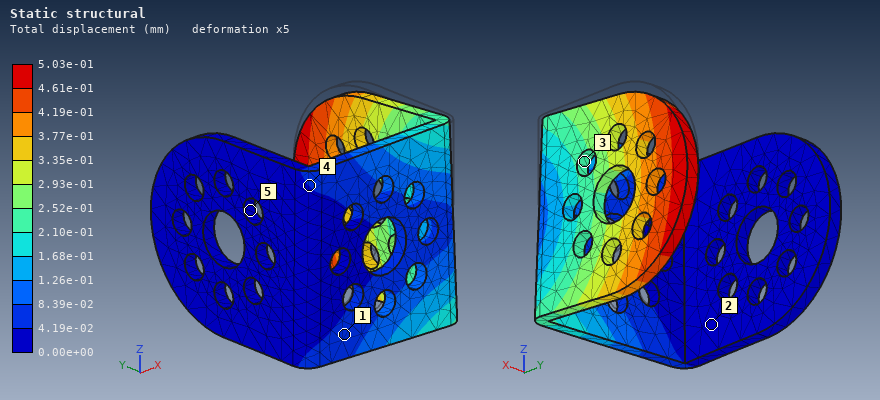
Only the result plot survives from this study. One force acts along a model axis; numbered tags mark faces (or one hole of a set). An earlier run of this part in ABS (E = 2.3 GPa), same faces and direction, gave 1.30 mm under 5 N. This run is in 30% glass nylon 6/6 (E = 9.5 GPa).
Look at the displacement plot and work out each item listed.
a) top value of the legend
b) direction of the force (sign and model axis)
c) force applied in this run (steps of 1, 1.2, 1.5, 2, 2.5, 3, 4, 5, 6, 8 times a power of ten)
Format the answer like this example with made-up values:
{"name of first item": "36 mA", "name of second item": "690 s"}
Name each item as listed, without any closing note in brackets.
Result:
{"top value of the legend": "5.03e-01 mm", "direction of the force": "-Z", "force applied in this run": "8 N"}
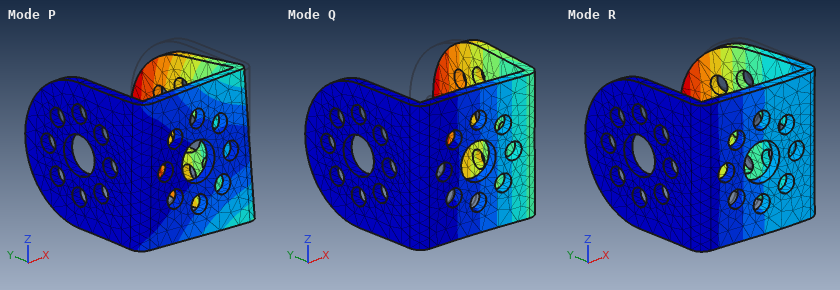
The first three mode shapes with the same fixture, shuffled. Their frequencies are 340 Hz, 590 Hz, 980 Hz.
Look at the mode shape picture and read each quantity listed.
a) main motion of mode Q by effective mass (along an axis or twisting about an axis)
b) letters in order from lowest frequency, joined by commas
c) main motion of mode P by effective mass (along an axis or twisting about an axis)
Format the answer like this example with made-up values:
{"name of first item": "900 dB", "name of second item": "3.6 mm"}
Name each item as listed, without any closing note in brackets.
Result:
{"main motion of mode Q by effective mass": "along Y", "letters in order from lowest frequency, joined by commas": "Q, P, R", "main motion of mode P by effective mass": "along Z"}
